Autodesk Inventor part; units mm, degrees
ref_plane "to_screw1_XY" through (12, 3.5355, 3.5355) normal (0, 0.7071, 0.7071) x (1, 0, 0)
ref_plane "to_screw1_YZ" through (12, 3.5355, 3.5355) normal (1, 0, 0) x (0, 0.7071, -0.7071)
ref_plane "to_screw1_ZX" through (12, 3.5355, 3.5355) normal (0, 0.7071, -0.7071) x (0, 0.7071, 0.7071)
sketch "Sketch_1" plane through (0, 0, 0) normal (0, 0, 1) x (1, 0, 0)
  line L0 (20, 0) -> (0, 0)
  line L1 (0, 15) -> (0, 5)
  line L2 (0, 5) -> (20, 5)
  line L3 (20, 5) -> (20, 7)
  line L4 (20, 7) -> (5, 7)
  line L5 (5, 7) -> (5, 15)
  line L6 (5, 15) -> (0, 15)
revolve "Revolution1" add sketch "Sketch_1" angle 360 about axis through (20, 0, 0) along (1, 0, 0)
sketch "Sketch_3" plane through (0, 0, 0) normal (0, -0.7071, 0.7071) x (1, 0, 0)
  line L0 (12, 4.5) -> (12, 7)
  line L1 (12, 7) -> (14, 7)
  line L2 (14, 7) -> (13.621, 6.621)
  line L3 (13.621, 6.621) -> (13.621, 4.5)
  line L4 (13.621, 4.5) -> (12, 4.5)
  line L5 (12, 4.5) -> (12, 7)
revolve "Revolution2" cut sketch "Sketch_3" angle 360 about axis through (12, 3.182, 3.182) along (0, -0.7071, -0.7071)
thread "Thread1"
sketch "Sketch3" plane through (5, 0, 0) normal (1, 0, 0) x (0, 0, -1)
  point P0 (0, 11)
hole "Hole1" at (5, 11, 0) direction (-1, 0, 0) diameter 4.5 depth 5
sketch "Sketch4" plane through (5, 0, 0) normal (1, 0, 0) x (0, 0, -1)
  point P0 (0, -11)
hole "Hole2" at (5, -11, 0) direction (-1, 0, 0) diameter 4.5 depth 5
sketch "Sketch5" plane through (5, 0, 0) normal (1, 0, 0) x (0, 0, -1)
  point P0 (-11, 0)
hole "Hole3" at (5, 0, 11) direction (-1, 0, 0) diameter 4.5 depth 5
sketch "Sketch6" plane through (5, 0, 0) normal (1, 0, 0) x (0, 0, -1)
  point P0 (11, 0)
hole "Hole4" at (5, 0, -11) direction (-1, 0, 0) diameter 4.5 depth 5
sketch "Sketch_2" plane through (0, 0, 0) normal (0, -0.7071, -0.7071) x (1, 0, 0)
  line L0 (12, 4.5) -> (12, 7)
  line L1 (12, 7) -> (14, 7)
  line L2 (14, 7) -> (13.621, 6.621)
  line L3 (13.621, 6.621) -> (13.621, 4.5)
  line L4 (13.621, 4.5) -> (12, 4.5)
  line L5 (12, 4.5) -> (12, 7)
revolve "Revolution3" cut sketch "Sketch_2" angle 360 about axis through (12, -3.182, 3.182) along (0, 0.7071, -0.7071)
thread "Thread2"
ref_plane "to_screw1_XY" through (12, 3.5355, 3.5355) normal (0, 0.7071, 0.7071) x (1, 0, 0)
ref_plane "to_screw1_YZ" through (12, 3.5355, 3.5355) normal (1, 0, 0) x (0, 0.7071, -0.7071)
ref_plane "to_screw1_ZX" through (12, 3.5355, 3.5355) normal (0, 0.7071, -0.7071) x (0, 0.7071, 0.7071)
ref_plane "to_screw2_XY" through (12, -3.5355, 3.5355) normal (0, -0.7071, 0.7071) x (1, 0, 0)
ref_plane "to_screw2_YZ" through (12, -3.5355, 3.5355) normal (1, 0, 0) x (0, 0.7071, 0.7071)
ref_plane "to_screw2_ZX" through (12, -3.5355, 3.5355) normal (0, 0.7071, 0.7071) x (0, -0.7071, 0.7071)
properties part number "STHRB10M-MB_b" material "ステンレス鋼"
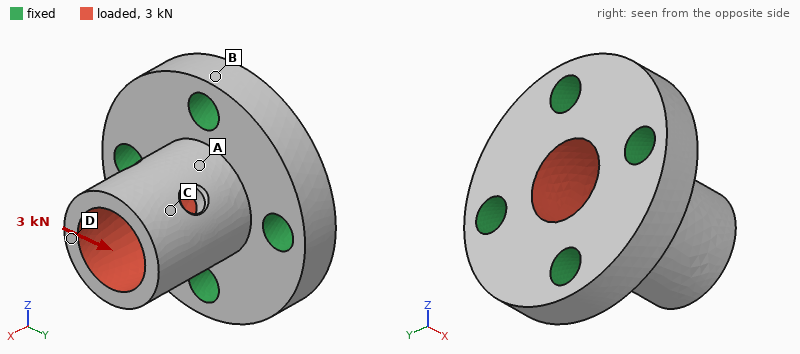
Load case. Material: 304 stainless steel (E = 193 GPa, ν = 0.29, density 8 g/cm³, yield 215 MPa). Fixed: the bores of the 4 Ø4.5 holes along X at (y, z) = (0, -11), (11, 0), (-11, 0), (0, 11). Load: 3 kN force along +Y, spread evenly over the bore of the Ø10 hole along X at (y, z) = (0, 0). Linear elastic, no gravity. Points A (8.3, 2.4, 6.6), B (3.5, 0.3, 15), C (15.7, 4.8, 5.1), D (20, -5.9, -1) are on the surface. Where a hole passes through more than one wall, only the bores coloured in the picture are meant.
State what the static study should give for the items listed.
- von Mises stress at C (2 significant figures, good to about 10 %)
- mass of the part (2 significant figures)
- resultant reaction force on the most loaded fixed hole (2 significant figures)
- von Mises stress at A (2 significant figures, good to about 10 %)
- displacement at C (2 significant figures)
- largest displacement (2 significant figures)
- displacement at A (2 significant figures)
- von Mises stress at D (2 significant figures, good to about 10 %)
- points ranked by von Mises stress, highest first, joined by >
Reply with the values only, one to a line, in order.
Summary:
37 MPa
31 g
1.5 kN
53 MPa
12 µm
16 µm
4.1 µm
23 MPa
A > C > D > B
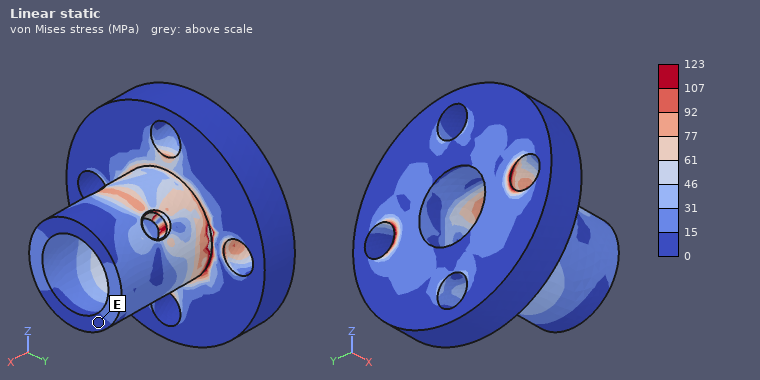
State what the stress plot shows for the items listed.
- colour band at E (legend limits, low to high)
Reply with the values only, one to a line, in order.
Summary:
0 to 15 MPa
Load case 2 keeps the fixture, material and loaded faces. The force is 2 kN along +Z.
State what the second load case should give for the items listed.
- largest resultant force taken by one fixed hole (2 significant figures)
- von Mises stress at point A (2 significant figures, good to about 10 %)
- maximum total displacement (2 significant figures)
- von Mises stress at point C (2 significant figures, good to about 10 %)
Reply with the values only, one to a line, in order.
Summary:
1000 N
30 MPa
11 µm
25 MPa
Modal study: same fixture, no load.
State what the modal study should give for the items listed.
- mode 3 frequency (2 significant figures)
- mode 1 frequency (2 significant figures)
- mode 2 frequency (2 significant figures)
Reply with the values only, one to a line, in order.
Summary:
37 kHz
24 kHz
24 kHz
